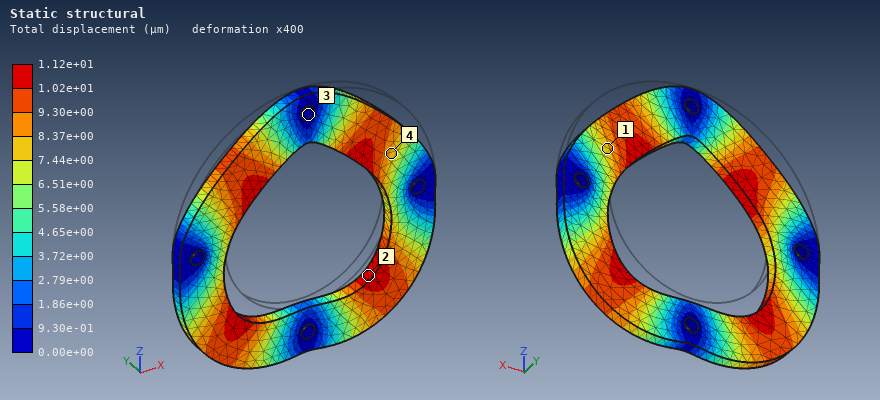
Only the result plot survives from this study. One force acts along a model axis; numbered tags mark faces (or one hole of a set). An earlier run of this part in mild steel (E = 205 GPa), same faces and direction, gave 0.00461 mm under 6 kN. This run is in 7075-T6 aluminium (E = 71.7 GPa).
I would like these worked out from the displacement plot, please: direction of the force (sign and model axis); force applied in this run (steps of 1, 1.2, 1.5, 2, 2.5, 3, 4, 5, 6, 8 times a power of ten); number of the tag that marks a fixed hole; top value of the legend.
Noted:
-Z
5 kN
3
1.12e+01 µm
